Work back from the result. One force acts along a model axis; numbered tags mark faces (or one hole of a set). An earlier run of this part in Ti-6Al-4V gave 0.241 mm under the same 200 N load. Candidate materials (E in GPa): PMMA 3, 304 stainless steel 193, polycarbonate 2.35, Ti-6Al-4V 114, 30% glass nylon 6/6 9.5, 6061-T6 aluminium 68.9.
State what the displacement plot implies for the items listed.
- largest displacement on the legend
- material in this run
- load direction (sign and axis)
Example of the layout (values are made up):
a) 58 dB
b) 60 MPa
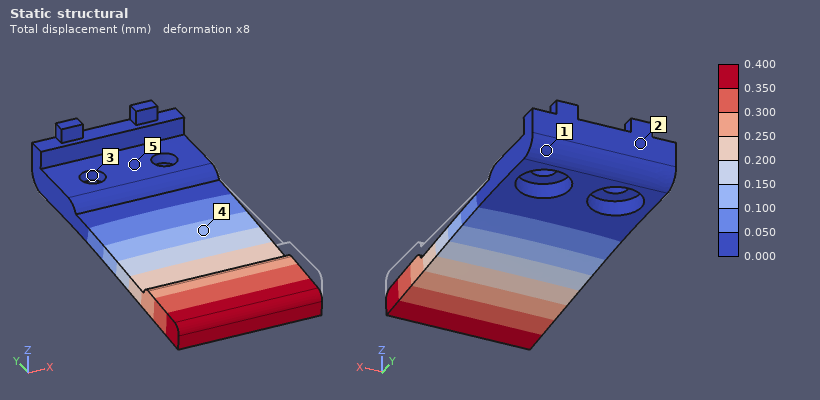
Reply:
a) 0.400 mm
b) 6061-T6 aluminium
c) -Z
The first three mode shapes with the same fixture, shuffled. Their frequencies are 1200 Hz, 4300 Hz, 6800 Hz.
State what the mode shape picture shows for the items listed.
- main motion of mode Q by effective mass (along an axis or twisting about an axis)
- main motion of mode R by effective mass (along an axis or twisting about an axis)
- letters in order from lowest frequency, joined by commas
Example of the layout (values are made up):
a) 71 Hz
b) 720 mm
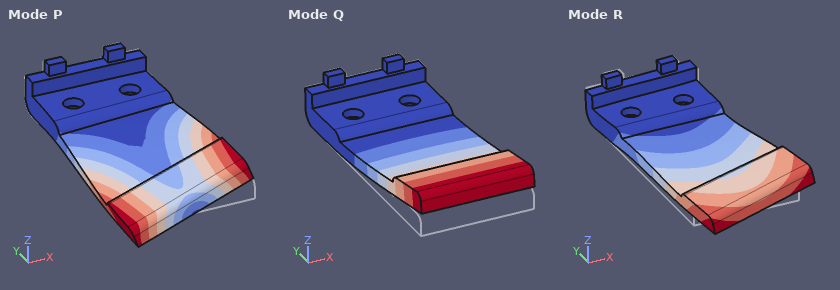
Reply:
a) along Z
b) along X
c) Q, P, R
